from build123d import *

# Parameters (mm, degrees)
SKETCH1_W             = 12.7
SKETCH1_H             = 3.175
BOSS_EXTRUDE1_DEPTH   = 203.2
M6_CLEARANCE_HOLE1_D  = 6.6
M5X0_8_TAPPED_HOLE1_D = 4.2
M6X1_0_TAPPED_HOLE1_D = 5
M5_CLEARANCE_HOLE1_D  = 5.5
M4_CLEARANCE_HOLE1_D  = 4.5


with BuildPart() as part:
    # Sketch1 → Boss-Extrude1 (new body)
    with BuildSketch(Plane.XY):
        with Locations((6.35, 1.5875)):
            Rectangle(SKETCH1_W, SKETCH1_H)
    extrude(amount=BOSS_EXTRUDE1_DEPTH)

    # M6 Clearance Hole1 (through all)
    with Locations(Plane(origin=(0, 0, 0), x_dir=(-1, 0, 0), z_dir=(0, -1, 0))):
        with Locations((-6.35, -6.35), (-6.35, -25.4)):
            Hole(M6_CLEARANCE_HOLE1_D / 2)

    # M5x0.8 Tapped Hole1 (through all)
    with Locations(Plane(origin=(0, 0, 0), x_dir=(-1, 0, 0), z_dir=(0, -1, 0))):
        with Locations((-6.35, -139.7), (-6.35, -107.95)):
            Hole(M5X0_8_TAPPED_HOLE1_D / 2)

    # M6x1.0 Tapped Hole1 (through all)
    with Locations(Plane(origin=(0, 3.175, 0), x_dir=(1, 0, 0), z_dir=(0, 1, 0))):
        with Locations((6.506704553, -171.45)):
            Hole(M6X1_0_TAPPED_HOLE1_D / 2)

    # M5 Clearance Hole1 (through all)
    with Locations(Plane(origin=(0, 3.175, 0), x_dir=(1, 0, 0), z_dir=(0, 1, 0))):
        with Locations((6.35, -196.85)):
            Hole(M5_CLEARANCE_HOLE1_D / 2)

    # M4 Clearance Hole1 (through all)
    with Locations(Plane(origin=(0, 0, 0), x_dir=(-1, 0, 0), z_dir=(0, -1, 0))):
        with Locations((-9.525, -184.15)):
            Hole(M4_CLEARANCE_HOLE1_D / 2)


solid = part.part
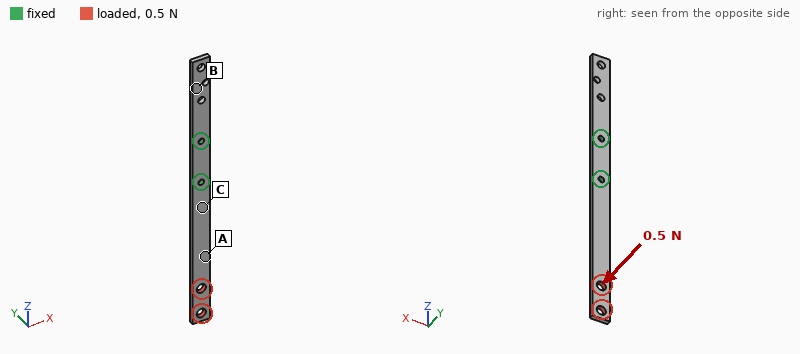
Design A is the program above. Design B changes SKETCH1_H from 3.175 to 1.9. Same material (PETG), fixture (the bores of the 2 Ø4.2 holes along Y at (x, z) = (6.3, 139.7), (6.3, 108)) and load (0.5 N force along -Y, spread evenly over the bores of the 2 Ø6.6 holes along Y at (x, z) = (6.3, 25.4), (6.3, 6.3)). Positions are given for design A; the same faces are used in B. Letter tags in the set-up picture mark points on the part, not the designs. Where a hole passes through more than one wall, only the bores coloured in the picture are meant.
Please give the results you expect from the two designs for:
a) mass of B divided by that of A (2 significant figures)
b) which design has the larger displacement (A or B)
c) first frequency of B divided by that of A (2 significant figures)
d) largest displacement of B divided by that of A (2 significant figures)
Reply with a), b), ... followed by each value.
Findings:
a) 0.60
b) B
c) 0.60
d) 4.6
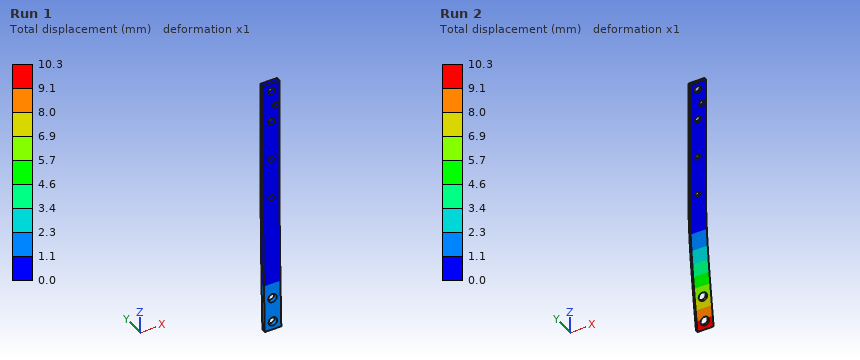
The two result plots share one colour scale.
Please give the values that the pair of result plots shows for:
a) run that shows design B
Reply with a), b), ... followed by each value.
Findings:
a) Run 2
